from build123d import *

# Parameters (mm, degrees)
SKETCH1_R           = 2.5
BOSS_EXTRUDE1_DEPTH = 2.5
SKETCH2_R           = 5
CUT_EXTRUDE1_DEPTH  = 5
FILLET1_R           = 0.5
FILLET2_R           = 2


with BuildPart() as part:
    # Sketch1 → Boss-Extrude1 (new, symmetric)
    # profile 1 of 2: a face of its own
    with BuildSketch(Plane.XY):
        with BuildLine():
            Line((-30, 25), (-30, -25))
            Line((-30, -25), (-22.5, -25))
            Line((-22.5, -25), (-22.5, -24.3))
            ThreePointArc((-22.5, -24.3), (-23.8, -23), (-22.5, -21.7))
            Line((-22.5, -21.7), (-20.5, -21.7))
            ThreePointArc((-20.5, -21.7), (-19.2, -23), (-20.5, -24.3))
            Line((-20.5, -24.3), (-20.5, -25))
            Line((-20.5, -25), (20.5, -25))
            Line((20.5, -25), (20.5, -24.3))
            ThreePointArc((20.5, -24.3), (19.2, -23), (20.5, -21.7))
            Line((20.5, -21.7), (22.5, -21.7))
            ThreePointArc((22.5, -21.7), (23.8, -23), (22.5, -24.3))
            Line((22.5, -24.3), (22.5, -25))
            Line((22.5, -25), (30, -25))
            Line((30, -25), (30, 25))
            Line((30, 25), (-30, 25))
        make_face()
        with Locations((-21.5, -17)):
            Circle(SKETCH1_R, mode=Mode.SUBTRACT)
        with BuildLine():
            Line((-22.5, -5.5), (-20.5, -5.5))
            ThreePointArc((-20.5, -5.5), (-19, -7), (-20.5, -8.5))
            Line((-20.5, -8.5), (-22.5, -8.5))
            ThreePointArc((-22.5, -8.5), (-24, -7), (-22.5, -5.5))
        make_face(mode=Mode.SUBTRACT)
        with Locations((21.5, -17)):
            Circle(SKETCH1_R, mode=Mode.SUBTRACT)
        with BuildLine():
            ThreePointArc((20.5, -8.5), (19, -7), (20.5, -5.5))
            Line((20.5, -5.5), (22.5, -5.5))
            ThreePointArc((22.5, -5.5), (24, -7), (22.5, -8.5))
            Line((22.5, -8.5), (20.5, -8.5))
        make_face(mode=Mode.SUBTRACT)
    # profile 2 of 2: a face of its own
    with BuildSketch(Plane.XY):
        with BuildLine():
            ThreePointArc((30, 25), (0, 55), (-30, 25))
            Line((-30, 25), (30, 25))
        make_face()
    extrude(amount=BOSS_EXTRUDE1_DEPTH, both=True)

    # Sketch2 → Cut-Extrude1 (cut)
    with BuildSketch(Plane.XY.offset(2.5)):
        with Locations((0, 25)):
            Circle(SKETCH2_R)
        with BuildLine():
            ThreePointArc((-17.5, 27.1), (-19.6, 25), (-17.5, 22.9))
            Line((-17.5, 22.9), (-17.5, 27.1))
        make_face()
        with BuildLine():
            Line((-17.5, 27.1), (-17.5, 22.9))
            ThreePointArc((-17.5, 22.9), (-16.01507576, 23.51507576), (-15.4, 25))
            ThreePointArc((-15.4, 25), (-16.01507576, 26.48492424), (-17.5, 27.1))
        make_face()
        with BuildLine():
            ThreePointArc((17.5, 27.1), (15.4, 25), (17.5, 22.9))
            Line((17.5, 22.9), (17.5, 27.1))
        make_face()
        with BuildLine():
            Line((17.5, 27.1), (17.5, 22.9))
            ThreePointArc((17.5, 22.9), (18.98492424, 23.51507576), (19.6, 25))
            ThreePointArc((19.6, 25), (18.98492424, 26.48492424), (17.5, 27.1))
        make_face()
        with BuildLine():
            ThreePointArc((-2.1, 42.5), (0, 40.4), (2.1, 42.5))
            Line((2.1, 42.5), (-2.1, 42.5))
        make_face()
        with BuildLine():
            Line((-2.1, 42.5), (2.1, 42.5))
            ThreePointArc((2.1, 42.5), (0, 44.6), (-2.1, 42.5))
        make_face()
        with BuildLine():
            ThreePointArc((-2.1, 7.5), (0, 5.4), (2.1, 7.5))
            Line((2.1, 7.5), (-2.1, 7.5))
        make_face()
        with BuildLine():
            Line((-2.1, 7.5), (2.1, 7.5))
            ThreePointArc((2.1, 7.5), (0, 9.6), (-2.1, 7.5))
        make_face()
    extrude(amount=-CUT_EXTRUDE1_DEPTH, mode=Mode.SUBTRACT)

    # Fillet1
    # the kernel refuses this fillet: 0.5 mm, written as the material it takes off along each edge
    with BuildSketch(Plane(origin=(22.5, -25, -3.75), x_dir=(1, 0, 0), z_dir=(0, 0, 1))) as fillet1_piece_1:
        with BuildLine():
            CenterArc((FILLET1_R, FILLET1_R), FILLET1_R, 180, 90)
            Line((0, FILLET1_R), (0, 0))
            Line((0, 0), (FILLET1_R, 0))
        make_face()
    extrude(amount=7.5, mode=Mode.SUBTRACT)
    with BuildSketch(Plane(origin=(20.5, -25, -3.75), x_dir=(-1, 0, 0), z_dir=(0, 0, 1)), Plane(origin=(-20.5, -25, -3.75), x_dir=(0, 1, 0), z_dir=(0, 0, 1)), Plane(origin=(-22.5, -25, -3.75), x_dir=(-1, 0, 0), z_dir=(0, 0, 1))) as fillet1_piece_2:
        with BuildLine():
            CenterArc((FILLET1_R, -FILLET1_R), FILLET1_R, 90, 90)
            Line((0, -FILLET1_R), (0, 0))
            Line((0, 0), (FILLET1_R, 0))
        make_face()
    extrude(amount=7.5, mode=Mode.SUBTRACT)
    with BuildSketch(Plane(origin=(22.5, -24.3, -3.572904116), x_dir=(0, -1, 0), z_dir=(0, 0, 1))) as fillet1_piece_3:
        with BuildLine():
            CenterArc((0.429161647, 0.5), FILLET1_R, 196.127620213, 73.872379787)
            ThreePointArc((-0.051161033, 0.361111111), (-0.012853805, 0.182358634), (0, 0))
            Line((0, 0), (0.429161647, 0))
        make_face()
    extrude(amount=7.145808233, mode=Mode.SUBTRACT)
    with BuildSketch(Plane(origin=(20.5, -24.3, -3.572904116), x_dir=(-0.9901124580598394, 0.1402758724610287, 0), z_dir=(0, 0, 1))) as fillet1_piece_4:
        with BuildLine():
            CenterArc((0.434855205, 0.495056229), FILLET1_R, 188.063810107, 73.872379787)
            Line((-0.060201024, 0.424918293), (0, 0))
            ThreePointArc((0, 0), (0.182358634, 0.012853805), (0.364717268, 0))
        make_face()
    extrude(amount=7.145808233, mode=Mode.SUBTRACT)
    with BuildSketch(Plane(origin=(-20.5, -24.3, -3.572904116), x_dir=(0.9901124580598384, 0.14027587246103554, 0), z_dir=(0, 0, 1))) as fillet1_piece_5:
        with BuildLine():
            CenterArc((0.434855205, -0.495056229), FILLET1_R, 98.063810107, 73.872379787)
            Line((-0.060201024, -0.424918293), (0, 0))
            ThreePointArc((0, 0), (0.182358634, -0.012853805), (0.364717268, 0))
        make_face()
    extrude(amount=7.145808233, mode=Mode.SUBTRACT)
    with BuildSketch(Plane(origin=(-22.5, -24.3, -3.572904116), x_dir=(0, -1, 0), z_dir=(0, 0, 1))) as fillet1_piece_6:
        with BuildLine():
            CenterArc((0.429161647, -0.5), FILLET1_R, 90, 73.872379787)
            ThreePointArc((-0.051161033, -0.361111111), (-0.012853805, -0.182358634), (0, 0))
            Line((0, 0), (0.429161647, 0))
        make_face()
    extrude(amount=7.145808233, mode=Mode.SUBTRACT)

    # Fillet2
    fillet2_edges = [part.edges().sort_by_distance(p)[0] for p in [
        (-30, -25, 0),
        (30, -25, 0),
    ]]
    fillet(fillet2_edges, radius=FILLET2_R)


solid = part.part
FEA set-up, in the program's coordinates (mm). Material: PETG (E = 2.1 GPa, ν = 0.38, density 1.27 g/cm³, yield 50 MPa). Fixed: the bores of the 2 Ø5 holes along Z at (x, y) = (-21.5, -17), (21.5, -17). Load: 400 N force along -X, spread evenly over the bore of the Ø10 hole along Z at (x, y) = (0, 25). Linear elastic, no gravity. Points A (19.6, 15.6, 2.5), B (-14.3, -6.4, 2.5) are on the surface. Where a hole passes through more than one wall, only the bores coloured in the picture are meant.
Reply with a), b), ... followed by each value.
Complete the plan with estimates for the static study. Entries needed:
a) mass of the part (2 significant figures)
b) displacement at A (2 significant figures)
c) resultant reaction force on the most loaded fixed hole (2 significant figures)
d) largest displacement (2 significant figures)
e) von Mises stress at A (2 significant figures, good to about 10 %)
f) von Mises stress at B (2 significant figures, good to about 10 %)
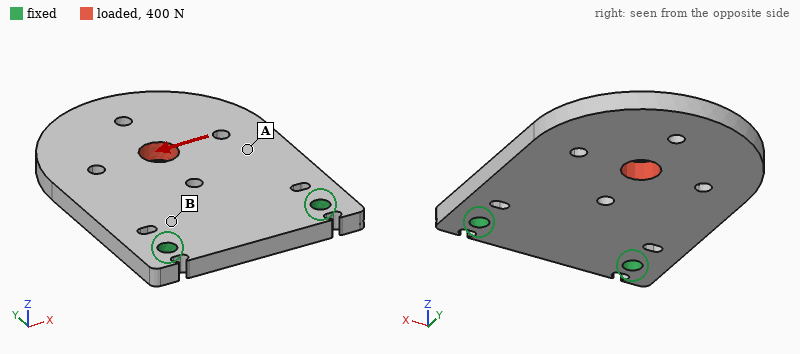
a) 27 g
b) 0.14 mm
c) 420 N
d) 0.25 mm
e) 2.2 MPa
f) 4.6 MPa
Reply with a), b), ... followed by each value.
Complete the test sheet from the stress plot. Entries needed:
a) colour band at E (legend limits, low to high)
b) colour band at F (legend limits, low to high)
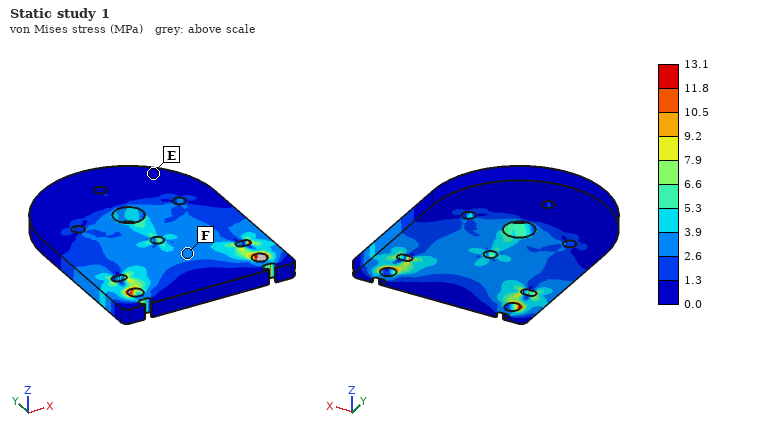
a) 0.0 to 1.3 MPa
b) 2.6 to 3.9 MPa
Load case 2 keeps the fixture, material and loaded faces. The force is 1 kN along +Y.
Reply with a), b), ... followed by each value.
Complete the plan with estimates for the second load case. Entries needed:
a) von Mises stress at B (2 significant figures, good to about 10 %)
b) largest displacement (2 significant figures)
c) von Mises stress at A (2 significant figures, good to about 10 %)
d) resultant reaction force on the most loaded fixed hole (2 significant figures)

a) 5.7 MPa
b) 0.15 mm
c) 2.4 MPa
d) 510 N
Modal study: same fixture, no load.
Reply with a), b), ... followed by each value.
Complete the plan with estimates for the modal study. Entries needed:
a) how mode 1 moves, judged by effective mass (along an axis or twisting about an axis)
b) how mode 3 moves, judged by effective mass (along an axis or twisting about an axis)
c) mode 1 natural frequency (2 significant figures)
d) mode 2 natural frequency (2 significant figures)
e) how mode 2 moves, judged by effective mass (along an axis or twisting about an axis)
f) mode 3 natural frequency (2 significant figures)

a) along Z
b) along Z
c) 220 Hz
d) 680 Hz
e) twisting about Y
f) 1200 Hz
